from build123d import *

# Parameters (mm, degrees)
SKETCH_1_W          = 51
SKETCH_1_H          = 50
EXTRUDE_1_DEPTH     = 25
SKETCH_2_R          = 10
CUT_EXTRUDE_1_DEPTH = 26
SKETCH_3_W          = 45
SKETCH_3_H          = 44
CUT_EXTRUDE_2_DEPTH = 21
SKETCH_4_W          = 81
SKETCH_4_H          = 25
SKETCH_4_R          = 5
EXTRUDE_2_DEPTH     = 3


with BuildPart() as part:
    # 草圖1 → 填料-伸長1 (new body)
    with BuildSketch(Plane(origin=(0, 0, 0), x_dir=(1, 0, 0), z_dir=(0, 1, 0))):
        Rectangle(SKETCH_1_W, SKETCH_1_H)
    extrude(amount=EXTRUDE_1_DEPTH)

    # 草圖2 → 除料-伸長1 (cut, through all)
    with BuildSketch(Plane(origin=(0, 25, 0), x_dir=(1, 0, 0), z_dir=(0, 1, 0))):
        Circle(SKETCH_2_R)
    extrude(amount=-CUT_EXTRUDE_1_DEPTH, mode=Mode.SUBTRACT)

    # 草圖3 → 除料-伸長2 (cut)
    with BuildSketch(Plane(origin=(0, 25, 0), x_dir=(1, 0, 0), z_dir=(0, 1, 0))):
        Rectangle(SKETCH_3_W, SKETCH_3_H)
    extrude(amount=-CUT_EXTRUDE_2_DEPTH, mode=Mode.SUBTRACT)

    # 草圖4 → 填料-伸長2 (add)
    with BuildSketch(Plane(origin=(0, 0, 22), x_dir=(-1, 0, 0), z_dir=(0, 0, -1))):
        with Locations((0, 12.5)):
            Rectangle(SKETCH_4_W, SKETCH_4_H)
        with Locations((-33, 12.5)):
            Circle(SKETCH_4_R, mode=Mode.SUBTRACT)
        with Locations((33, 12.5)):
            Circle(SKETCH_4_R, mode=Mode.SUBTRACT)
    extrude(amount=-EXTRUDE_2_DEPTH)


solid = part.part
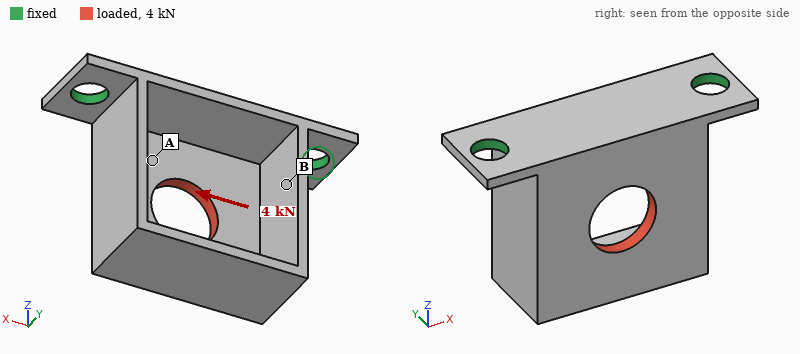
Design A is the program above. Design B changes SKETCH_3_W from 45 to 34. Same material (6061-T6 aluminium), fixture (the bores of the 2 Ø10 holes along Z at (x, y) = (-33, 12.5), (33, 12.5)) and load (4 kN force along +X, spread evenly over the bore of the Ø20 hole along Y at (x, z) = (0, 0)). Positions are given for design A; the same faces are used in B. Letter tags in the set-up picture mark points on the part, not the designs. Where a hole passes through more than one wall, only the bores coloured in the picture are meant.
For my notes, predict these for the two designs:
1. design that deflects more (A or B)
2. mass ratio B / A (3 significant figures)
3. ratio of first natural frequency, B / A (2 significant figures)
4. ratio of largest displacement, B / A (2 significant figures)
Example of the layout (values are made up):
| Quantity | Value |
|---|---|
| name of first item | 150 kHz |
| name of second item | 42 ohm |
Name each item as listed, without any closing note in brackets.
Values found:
| Quantity | Value |
|---|---|
| design that deflects more | A |
| mass ratio B / A | 1.45 |
| ratio of first natural frequency, B / A | 0.90 |
| ratio of largest displacement, B / A | 0.34 |
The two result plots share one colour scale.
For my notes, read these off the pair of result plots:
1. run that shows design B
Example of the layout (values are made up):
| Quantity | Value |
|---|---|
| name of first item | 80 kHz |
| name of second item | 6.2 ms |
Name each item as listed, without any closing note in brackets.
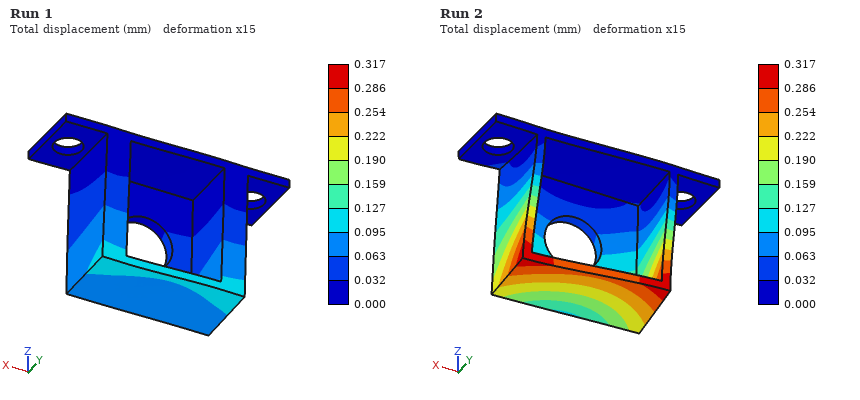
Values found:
| Quantity | Value |
|---|---|
| run that shows design B | Run 1 |
